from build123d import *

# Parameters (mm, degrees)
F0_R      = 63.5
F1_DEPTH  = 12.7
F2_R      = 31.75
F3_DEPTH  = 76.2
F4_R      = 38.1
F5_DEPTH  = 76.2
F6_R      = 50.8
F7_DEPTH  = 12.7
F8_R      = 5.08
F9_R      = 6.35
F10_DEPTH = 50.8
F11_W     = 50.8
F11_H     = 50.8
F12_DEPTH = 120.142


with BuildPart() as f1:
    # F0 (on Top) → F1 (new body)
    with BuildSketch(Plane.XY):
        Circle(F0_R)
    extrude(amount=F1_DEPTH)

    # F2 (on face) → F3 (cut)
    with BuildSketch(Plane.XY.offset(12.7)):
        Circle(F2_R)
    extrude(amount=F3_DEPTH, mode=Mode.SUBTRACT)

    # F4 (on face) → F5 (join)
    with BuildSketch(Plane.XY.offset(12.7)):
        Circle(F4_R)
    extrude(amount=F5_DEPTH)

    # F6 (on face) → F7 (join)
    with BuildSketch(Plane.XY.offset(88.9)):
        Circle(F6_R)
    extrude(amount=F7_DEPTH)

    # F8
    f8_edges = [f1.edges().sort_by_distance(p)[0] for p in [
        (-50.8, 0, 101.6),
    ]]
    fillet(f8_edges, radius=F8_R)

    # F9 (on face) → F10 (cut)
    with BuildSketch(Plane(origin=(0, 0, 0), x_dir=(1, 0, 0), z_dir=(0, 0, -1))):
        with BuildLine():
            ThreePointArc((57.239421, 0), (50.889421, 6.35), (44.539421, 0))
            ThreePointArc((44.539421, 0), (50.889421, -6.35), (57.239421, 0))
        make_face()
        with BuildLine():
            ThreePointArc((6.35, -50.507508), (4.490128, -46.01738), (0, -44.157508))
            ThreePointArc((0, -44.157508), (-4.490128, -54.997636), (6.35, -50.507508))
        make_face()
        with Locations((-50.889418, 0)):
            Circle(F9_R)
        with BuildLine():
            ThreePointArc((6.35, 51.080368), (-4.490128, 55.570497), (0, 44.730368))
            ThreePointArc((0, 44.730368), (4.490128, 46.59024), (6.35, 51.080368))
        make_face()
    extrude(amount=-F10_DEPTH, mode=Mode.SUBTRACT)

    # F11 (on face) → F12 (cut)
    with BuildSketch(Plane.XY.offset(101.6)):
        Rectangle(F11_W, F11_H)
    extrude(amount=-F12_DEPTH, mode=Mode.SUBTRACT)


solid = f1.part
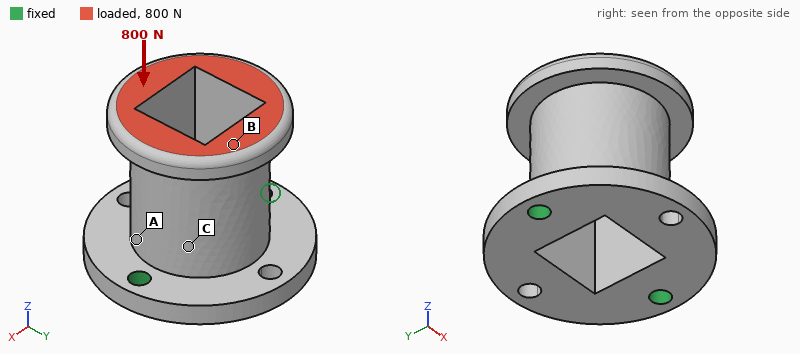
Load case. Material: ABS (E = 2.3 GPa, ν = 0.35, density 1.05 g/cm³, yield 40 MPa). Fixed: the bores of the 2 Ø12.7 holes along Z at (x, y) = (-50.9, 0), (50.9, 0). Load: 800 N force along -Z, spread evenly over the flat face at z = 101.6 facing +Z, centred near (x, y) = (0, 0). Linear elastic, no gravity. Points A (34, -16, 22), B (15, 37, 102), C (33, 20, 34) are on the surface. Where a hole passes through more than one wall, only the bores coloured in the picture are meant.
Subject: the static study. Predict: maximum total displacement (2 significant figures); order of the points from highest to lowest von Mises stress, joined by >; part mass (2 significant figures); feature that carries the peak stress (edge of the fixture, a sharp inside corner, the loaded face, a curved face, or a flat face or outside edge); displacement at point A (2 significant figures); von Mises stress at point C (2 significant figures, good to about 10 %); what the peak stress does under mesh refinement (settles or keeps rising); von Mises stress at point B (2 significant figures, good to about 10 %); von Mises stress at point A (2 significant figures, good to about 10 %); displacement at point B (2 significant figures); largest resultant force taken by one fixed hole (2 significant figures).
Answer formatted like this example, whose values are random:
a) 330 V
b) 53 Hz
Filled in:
a) 67 µm
b) A > C > B
c) 360 g
d) edge of the fixture
e) 39 µm
f) 0.79 MPa
g) keeps rising
h) 0.35 MPa
i) 1.3 MPa
j) 60 µm
k) 410 N
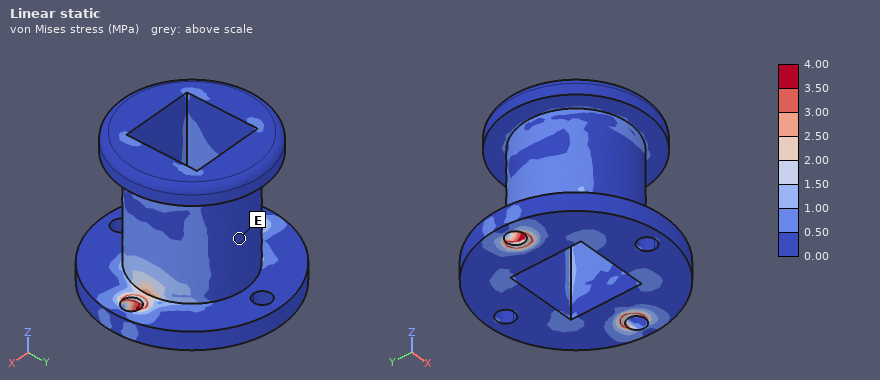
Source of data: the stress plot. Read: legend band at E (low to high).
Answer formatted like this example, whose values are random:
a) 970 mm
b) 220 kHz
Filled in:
a) 0.00 to 0.50 MPa
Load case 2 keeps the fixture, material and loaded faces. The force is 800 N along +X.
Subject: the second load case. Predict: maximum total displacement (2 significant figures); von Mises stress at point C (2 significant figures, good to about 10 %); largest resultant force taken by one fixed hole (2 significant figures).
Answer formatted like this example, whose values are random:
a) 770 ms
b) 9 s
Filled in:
a) 0.41 mm
b) 2.1 MPa
c) 1.0 kN
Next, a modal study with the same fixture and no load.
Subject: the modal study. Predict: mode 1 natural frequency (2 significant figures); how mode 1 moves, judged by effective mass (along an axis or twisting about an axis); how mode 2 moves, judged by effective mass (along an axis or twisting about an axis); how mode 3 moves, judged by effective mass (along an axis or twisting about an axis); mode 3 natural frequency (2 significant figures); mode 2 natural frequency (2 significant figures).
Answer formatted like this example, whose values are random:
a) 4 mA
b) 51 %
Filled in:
a) 270 Hz
b) along Y
c) along X
d) along Z
e) 1100 Hz
f) 710 Hz
